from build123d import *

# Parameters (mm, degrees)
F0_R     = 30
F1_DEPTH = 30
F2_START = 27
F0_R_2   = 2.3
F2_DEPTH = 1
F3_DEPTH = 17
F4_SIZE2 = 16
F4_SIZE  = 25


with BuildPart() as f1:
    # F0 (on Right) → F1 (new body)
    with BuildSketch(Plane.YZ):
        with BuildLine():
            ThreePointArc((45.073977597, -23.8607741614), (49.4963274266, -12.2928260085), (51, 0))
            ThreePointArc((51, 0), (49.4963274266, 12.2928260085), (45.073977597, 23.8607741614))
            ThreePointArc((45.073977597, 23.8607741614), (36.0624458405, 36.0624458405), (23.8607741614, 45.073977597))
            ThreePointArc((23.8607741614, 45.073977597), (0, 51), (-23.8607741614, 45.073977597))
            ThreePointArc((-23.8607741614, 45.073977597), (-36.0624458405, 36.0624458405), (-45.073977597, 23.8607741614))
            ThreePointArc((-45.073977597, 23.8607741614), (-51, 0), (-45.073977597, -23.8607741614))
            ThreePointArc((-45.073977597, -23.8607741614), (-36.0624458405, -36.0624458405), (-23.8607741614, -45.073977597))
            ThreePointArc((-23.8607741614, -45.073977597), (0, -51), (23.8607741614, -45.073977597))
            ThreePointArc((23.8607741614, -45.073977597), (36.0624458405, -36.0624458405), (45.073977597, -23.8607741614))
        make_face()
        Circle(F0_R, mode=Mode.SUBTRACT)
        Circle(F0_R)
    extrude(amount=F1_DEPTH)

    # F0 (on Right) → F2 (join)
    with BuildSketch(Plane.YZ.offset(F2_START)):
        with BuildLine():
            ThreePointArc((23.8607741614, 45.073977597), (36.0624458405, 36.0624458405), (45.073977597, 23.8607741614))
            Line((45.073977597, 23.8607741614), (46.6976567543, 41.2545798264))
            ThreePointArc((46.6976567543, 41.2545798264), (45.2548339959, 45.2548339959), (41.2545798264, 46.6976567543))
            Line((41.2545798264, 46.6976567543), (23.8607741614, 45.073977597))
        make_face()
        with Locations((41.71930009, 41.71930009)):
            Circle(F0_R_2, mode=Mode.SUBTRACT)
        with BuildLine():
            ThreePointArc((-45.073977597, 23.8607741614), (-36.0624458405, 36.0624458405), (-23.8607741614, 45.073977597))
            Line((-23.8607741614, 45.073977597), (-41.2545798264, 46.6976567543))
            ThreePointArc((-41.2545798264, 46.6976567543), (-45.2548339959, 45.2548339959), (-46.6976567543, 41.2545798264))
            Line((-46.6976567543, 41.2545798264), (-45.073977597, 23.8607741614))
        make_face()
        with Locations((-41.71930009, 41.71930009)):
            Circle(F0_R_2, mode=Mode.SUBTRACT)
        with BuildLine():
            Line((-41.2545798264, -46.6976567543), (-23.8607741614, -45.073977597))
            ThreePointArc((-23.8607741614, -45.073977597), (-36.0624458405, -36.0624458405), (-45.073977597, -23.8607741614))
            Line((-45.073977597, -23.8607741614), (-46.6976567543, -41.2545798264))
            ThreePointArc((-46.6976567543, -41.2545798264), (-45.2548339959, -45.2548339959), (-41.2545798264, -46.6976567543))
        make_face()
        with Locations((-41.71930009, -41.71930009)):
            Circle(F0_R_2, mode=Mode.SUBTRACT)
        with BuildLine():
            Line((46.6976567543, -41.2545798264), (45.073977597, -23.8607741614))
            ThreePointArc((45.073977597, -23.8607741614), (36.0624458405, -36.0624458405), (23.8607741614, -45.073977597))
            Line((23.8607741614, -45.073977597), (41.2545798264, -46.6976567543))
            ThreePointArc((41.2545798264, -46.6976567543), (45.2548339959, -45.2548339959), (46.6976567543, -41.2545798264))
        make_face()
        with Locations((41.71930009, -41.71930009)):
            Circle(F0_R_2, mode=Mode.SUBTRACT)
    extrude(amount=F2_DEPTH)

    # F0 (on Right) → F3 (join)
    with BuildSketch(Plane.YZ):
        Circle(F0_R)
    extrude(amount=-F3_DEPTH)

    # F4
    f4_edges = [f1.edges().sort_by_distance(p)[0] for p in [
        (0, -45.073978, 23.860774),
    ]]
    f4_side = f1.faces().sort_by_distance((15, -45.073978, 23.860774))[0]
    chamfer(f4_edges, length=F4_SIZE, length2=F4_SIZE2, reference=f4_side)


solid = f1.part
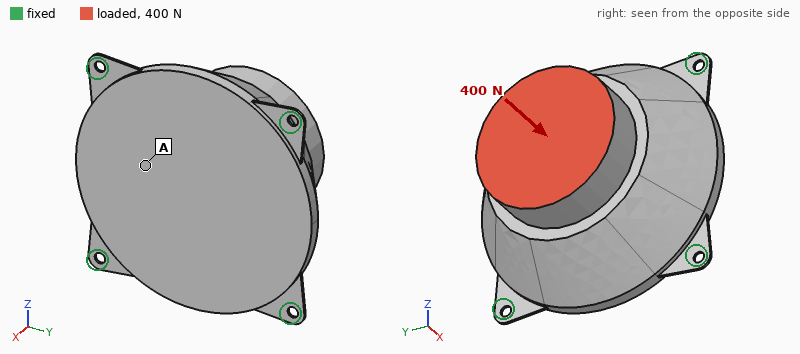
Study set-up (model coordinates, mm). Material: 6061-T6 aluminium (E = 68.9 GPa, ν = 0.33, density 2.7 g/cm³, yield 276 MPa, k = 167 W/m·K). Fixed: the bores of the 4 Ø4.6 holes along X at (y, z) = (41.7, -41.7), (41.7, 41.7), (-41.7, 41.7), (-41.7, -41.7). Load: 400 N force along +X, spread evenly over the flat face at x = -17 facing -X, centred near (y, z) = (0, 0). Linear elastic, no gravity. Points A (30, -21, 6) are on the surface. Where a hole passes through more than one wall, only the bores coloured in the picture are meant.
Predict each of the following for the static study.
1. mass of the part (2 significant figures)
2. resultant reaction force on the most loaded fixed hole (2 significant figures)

640 g
100 N
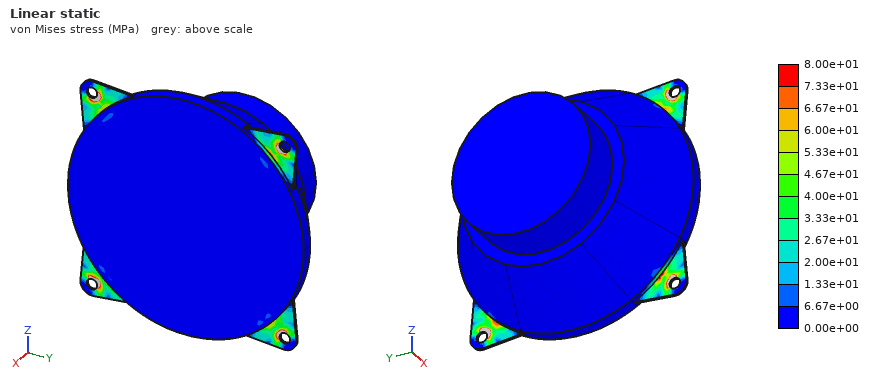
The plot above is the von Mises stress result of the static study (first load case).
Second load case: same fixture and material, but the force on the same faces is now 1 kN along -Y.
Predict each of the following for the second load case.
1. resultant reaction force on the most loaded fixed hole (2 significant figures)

400 N
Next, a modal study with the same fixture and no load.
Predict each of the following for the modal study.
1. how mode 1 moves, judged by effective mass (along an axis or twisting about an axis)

along X
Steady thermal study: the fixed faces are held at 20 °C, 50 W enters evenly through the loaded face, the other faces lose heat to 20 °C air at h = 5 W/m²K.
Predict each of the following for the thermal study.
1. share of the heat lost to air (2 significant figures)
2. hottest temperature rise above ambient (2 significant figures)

8.6 %
41 K
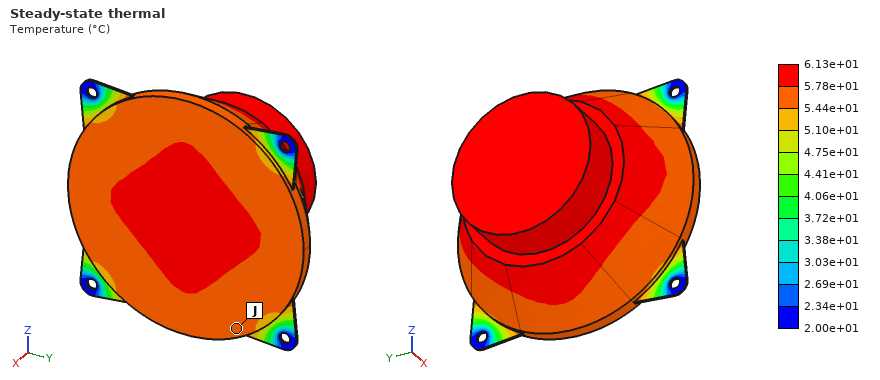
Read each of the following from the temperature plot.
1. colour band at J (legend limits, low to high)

5.44e+01 to 5.78e+01 °C
